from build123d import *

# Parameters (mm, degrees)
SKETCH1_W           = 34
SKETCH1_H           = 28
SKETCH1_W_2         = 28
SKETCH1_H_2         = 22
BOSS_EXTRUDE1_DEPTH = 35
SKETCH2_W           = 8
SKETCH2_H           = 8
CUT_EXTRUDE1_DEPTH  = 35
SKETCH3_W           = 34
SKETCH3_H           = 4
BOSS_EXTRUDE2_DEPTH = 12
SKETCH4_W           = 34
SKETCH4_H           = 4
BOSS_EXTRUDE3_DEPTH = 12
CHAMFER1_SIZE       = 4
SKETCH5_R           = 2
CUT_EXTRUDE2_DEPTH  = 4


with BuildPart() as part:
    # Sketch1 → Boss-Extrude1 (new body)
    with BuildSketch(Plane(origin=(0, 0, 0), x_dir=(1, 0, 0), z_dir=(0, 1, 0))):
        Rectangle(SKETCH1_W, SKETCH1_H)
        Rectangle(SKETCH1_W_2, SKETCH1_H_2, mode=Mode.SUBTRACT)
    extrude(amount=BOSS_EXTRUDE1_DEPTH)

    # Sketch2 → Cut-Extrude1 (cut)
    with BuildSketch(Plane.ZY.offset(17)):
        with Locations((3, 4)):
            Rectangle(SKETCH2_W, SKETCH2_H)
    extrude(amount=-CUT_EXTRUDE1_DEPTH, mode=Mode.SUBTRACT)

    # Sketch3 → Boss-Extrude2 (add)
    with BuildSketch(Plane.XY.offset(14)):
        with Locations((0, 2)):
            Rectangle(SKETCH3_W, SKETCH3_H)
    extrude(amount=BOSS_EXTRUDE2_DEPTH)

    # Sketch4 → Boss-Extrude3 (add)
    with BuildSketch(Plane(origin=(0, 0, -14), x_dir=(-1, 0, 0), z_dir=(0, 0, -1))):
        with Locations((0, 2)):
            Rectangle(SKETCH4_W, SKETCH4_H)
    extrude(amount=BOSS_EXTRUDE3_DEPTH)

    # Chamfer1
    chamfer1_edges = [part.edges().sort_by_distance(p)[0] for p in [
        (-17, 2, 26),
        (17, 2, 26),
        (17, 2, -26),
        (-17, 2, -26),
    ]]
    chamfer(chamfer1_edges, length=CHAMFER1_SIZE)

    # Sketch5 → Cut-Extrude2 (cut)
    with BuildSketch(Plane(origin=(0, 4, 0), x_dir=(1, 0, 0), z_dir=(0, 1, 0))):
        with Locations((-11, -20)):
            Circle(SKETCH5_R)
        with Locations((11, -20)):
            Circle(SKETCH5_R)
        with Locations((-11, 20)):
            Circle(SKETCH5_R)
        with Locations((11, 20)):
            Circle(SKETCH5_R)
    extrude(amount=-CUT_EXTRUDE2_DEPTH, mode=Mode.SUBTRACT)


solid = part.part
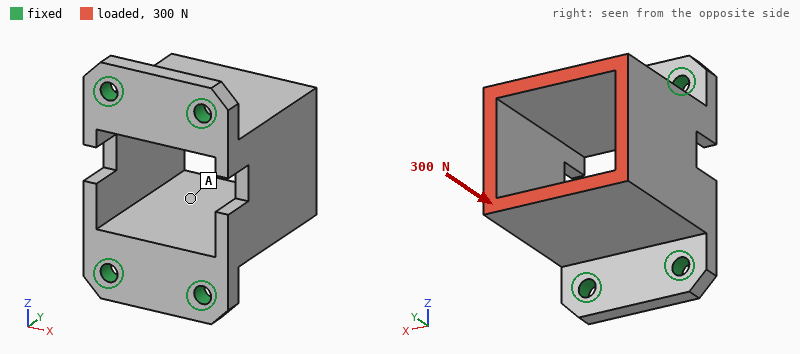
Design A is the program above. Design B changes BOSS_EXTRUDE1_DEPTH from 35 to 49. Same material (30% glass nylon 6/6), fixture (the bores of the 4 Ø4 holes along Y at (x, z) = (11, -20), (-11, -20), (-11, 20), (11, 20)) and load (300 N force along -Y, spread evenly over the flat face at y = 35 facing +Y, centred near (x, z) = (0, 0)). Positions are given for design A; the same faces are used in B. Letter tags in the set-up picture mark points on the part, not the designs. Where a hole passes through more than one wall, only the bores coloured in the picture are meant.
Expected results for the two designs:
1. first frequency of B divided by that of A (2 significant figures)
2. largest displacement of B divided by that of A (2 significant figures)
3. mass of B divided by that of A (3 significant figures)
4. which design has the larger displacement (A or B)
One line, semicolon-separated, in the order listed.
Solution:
0.64; 1.1; 1.33; B
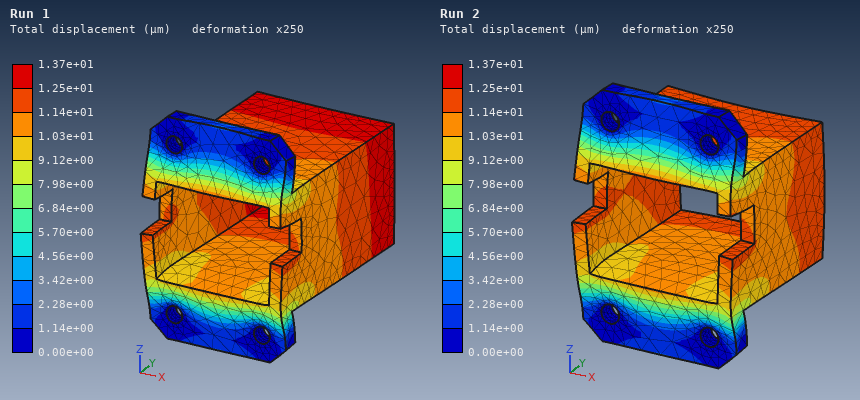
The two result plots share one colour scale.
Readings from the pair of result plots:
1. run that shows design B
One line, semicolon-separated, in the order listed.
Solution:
Run 1
